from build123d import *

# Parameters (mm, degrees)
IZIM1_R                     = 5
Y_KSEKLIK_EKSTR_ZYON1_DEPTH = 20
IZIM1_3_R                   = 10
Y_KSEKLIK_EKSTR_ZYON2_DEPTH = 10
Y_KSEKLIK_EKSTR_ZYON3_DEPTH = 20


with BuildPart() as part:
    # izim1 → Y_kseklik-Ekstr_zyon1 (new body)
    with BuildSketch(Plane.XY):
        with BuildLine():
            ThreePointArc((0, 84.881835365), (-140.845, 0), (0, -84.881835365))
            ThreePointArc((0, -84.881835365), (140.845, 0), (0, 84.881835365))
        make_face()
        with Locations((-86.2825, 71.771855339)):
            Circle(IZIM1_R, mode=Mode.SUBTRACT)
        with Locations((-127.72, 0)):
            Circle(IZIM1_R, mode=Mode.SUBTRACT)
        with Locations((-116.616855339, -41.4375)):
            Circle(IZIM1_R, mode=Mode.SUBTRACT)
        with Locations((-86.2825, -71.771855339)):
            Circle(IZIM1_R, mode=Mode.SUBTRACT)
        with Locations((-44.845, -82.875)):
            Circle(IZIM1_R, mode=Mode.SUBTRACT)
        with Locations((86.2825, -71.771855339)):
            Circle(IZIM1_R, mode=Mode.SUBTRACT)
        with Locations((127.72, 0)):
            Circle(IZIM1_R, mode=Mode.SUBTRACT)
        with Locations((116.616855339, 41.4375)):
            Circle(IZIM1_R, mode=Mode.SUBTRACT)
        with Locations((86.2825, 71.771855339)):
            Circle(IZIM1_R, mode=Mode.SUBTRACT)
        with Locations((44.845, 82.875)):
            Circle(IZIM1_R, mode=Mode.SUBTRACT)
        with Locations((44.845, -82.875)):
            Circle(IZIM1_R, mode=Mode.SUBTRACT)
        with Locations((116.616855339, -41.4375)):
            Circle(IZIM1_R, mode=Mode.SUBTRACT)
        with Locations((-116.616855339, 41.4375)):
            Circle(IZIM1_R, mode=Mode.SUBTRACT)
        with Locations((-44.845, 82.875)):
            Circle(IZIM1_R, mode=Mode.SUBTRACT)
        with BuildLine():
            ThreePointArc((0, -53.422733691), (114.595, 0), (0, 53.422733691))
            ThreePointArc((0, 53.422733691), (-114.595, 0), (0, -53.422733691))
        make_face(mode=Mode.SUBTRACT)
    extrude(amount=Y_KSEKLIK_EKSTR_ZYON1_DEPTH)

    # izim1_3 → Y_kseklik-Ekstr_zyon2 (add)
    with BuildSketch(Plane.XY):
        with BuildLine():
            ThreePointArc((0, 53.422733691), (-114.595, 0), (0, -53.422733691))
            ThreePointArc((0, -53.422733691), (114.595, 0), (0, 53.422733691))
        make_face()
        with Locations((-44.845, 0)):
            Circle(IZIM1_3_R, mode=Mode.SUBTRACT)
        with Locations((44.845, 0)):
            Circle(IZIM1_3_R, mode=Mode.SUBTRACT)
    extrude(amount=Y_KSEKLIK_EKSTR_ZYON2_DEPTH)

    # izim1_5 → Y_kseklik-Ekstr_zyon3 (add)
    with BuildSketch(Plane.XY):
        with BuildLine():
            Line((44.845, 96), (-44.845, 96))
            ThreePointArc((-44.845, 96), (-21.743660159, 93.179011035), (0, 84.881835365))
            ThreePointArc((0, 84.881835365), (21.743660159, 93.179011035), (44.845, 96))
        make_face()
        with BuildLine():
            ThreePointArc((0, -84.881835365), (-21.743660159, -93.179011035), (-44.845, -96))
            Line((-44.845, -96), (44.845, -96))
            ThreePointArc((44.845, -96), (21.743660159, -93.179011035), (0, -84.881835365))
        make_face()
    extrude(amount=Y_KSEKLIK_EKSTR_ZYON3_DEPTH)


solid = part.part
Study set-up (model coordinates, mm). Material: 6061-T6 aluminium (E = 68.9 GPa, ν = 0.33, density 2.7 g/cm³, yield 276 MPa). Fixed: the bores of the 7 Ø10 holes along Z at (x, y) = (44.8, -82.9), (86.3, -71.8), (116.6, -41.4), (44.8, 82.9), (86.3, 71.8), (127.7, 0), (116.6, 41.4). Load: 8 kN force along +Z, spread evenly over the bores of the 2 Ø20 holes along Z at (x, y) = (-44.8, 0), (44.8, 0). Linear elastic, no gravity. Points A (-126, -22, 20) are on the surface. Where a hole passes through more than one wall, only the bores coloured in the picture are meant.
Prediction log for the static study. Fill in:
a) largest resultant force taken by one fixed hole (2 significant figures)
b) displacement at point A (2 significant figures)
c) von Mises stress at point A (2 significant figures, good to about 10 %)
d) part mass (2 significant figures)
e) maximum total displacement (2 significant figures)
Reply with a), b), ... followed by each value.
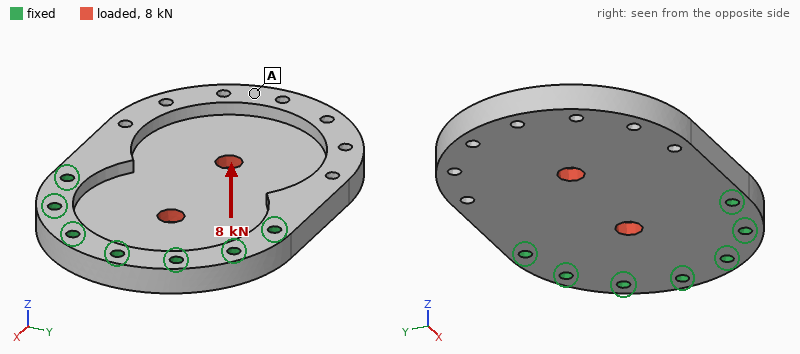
a) 5.9 kN
b) 0.70 mm
c) 17 MPa
d) 1.7 kg
e) 0.77 mm
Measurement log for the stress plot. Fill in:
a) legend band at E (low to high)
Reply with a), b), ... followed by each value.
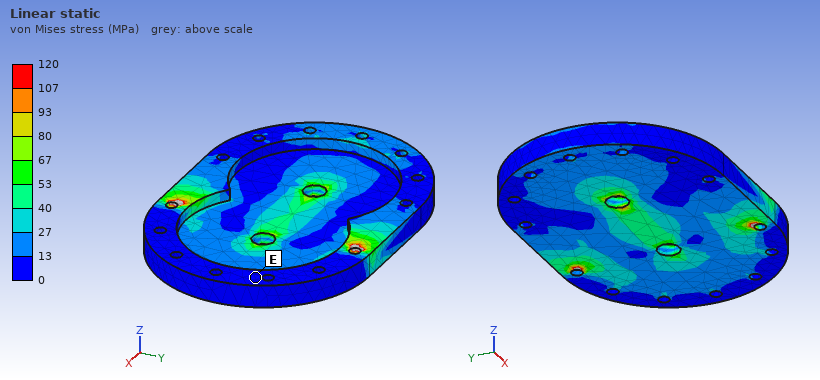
a) 0 to 13 MPa
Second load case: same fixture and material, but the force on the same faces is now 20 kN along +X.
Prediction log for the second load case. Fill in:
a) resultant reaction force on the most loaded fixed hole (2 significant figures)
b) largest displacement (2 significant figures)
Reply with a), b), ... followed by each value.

a) 4.1 kN
b) 0.10 mm
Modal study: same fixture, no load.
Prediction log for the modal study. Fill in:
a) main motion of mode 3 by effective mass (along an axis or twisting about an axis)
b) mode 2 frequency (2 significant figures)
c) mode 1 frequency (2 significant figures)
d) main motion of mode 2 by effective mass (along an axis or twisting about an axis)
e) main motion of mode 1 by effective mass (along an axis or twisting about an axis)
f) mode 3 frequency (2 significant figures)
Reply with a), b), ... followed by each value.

a) along Z
b) 1100 Hz
c) 430 Hz
d) twisting about X
e) along Z
f) 2000 Hz
